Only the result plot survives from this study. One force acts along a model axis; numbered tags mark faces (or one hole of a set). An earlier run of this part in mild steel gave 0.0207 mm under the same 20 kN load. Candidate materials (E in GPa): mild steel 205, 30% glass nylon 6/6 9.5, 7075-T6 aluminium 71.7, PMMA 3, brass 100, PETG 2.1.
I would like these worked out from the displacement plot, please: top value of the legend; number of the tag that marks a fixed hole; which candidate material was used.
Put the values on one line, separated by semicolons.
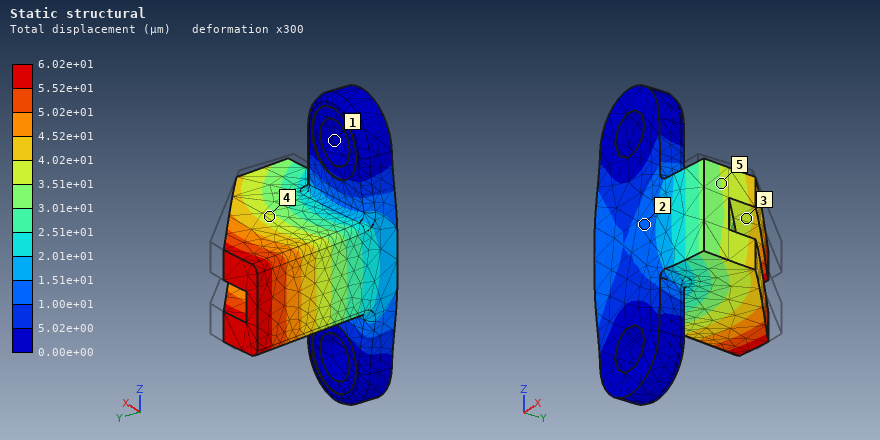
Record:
6.02e+01 µm; 1; 7075-T6 aluminium
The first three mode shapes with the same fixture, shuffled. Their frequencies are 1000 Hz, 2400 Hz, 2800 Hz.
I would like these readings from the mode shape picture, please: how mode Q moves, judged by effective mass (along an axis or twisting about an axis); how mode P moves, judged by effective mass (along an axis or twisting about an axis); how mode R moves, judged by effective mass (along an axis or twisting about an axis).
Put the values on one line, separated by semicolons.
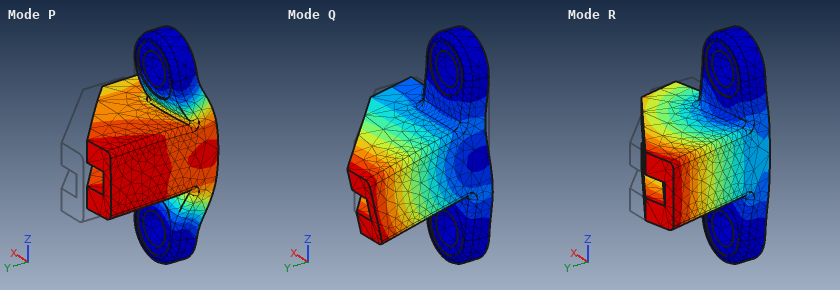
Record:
along Z; along Y; along X
